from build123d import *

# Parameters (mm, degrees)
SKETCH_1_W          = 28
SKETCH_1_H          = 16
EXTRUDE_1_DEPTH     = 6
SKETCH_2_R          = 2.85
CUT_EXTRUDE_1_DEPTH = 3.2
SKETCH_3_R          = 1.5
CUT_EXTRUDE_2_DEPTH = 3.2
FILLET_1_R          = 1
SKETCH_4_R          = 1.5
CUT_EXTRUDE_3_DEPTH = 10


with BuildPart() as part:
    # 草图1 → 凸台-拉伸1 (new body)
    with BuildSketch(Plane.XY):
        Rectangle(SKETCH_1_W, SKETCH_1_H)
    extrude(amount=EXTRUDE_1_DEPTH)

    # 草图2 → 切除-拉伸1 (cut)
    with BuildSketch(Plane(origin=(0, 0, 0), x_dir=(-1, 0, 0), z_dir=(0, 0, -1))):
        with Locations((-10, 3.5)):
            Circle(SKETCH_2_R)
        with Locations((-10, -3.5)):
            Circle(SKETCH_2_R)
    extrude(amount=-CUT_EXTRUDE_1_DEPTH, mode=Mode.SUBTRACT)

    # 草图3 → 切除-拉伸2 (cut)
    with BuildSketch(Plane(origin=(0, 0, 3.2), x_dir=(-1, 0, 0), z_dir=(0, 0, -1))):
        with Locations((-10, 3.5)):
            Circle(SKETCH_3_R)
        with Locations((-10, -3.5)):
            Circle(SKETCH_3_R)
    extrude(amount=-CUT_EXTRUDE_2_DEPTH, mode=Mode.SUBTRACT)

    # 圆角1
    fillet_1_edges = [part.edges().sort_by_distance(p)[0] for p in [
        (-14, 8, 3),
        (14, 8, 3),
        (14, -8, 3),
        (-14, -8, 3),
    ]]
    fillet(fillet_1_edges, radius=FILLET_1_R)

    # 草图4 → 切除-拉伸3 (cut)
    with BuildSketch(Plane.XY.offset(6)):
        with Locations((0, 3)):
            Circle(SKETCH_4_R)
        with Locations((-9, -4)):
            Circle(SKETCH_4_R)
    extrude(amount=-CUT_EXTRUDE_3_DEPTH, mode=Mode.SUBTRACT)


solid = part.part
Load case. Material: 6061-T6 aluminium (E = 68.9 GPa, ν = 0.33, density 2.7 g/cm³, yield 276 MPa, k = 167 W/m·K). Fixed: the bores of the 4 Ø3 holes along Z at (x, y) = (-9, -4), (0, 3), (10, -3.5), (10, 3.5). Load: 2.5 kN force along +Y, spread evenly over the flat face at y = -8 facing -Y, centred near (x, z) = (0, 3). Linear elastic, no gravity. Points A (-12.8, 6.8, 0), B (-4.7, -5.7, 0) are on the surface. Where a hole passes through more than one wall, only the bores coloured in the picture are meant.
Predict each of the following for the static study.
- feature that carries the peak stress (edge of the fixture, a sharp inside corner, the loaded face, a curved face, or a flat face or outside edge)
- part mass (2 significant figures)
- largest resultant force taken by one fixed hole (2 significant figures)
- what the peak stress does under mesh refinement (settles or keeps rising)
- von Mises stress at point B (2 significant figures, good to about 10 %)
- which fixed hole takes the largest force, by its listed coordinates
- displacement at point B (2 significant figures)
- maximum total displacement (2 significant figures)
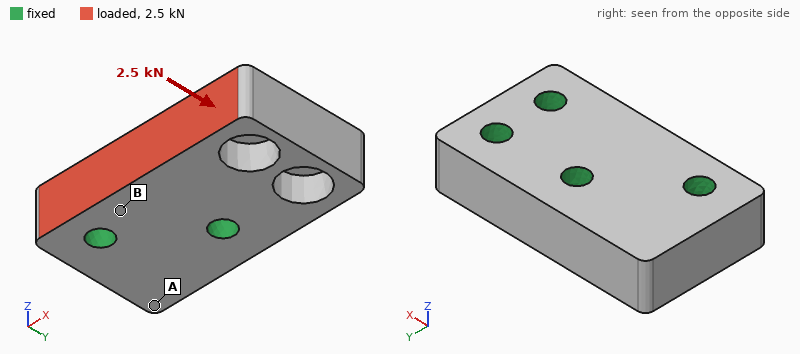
edge of the fixture
6.5 g
930 N
keeps rising
13 MPa
(-9, -4)
1.5 µm
6.6 µm
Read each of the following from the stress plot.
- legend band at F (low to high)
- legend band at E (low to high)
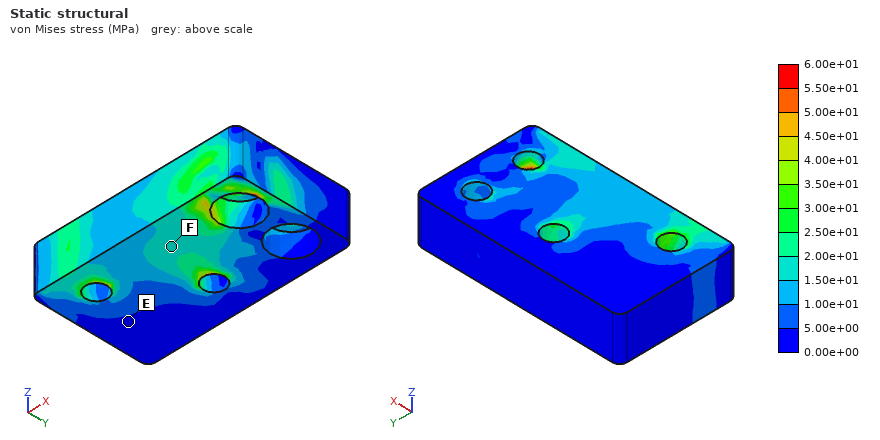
1.50e+01 to 2.00e+01 MPa
0.00e+00 to 5.00e+00 MPa
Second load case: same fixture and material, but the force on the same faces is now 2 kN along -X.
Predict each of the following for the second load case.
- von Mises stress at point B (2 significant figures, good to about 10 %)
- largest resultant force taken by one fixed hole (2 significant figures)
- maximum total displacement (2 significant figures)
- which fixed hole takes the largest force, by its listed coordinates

23 MPa
1.2 kN
5.7 µm
(-9, -4)
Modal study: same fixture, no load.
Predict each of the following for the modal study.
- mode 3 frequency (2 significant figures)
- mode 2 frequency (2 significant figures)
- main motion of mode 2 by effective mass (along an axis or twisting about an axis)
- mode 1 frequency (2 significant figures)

81 kHz
62 kHz
along Z
44 kHz
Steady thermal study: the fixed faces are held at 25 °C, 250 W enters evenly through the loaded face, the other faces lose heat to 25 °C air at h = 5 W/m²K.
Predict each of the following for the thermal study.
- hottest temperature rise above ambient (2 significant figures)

74 K
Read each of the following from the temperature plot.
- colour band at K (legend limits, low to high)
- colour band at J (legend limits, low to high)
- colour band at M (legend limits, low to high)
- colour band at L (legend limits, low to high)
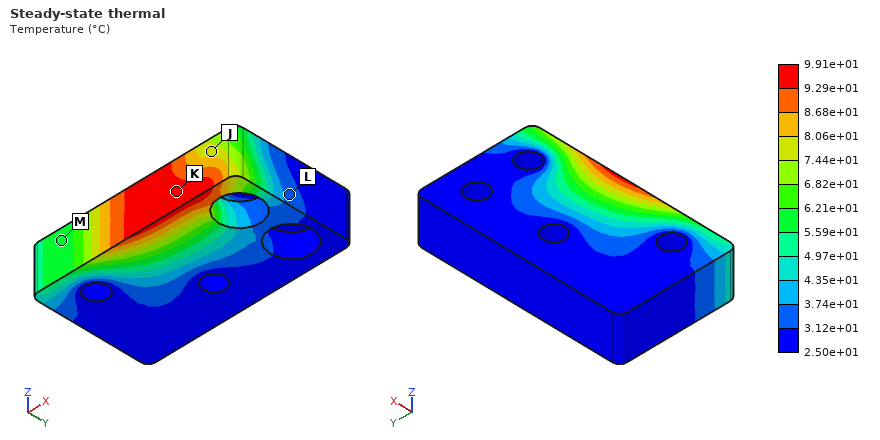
9.29e+01 to 9.91e+01 °C
7.44e+01 to 8.06e+01 °C
5.59e+01 to 6.21e+01 °C
3.12e+01 to 3.74e+01 °C
